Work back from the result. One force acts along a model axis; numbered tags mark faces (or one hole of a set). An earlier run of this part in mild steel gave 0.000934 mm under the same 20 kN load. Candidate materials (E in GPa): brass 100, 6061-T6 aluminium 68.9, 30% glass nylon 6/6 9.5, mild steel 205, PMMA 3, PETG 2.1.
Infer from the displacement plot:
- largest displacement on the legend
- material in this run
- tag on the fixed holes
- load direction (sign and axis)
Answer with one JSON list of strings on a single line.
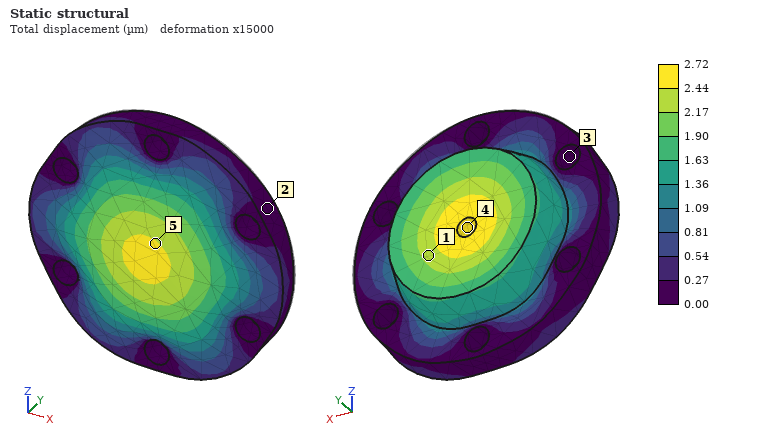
["2.72 µm", "6061-T6 aluminium", "3", "-Y"]
